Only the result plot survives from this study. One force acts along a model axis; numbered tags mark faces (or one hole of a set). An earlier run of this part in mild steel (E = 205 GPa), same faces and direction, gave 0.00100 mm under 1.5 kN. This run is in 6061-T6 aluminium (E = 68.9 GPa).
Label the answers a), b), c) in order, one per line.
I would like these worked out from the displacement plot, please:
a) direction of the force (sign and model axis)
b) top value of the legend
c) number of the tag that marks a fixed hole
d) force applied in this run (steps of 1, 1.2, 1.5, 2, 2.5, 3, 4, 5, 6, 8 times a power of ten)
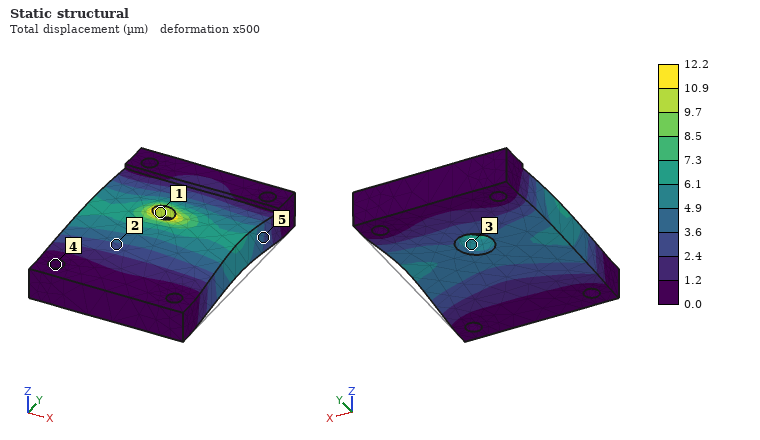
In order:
a) -X
b) 12.2 µm
c) 4
d) 6 kN
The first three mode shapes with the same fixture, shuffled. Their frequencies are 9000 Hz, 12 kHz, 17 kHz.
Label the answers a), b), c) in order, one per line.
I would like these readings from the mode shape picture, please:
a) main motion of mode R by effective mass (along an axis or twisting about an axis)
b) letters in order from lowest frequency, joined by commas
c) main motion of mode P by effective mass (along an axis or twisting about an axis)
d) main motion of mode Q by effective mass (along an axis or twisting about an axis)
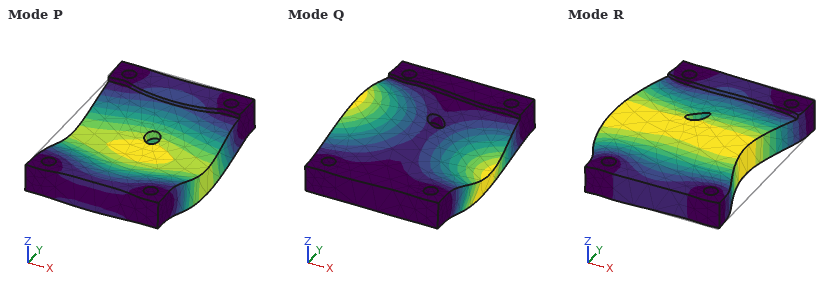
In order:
a) along X
b) P, Q, R
c) along Z
d) twisting about Y
